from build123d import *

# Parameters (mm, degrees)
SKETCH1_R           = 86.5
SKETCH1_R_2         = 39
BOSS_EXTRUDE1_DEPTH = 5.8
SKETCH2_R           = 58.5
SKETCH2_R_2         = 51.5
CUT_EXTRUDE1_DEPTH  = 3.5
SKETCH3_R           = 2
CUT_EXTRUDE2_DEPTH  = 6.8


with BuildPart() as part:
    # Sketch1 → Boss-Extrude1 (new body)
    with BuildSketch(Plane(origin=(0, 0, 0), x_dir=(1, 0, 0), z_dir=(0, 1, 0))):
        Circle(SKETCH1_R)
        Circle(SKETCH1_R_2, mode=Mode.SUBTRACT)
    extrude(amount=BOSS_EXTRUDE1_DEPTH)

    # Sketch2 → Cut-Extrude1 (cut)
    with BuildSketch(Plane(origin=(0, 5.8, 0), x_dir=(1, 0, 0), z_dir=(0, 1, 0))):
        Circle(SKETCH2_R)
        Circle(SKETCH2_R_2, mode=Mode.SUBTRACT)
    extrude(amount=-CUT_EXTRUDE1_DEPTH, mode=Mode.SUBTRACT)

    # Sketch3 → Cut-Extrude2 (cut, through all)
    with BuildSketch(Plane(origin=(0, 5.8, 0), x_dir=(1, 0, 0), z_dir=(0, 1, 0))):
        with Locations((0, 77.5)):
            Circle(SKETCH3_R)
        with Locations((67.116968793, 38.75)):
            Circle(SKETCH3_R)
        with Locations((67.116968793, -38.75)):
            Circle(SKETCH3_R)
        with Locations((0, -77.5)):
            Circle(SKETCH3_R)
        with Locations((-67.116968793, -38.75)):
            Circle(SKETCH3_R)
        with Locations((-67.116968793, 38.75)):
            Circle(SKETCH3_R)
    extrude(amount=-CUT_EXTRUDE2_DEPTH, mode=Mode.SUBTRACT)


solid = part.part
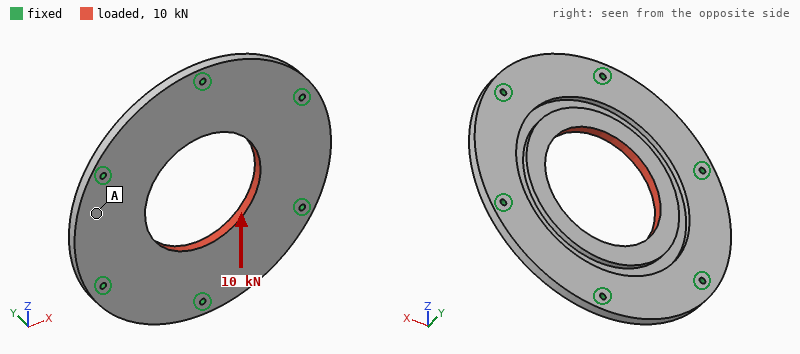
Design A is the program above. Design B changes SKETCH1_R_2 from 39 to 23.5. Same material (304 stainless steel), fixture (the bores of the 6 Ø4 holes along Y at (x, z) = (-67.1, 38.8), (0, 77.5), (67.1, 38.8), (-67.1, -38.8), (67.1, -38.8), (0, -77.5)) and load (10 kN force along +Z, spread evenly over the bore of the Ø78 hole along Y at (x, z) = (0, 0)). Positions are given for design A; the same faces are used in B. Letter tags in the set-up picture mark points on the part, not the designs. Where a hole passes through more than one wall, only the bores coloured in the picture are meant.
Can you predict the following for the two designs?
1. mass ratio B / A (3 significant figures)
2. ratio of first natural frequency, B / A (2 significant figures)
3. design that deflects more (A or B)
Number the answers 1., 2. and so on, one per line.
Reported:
1. 1.18
2. 0.71
3. B
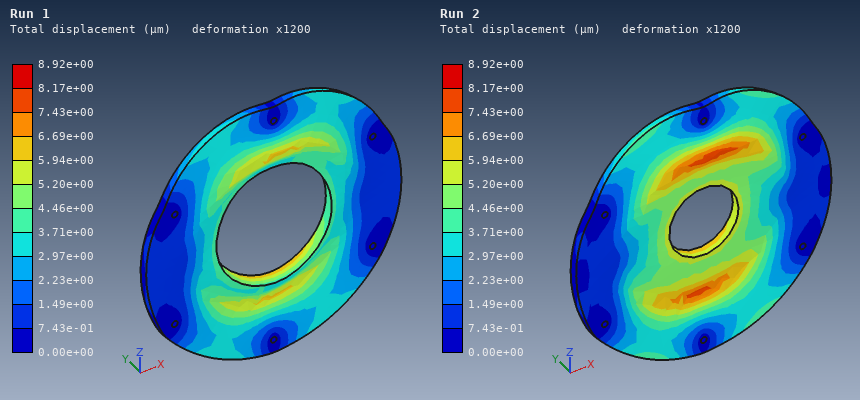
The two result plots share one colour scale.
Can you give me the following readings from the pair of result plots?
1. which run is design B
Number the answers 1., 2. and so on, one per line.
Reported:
1. Run 2
